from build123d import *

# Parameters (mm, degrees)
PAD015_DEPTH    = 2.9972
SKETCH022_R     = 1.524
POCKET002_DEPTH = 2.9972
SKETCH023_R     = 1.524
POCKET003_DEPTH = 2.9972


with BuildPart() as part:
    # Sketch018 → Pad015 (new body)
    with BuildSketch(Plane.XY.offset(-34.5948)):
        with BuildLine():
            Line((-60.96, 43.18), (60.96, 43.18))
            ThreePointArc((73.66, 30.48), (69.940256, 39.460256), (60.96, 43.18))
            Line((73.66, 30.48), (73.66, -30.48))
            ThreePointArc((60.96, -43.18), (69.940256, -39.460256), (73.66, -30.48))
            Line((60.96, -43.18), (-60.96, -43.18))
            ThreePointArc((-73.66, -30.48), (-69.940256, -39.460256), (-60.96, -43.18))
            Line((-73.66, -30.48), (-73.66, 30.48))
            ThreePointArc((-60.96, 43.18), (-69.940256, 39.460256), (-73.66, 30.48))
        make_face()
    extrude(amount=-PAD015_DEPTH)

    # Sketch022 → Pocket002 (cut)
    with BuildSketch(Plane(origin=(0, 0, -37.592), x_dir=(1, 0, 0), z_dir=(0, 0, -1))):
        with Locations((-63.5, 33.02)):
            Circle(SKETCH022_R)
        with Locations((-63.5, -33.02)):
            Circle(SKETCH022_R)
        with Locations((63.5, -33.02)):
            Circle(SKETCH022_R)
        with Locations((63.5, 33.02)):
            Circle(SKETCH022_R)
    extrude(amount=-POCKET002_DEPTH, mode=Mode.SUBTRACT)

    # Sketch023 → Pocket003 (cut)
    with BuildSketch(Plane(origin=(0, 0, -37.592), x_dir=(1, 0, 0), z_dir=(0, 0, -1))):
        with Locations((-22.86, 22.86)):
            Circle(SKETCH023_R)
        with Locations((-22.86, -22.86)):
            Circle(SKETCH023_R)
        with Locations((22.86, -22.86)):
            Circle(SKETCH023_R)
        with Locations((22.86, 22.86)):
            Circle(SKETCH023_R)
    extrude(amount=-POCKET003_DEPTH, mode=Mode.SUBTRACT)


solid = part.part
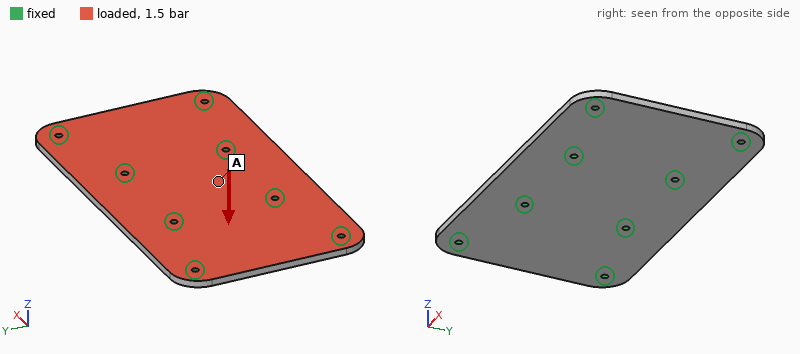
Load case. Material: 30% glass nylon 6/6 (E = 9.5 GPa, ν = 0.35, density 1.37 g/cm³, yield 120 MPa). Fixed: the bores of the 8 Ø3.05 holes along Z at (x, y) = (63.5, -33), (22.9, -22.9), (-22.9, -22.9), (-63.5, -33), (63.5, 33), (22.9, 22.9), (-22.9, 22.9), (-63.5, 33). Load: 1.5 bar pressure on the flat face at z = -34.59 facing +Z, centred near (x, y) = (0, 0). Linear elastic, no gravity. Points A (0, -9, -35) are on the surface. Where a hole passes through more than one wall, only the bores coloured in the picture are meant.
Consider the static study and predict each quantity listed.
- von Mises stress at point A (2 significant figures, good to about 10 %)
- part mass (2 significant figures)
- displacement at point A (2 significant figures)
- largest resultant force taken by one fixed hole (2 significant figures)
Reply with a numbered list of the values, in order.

1. 6.1 MPa
2. 51 g
3. 0.13 mm
4. 290 N
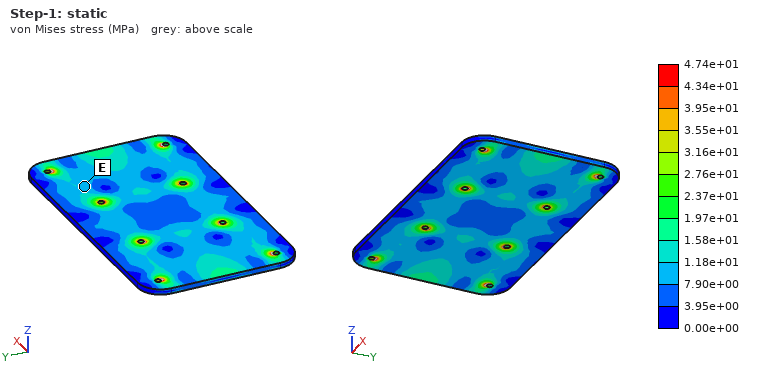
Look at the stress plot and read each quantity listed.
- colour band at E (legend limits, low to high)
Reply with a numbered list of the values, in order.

1. 7.90e+00 to 1.18e+01 MPa
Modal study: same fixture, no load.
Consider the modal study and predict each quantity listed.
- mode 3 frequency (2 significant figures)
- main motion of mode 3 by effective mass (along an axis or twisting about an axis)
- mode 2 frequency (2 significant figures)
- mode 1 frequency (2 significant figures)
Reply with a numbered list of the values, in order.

1. 2400 Hz
2. along Z
3. 1900 Hz
4. 1900 Hz
